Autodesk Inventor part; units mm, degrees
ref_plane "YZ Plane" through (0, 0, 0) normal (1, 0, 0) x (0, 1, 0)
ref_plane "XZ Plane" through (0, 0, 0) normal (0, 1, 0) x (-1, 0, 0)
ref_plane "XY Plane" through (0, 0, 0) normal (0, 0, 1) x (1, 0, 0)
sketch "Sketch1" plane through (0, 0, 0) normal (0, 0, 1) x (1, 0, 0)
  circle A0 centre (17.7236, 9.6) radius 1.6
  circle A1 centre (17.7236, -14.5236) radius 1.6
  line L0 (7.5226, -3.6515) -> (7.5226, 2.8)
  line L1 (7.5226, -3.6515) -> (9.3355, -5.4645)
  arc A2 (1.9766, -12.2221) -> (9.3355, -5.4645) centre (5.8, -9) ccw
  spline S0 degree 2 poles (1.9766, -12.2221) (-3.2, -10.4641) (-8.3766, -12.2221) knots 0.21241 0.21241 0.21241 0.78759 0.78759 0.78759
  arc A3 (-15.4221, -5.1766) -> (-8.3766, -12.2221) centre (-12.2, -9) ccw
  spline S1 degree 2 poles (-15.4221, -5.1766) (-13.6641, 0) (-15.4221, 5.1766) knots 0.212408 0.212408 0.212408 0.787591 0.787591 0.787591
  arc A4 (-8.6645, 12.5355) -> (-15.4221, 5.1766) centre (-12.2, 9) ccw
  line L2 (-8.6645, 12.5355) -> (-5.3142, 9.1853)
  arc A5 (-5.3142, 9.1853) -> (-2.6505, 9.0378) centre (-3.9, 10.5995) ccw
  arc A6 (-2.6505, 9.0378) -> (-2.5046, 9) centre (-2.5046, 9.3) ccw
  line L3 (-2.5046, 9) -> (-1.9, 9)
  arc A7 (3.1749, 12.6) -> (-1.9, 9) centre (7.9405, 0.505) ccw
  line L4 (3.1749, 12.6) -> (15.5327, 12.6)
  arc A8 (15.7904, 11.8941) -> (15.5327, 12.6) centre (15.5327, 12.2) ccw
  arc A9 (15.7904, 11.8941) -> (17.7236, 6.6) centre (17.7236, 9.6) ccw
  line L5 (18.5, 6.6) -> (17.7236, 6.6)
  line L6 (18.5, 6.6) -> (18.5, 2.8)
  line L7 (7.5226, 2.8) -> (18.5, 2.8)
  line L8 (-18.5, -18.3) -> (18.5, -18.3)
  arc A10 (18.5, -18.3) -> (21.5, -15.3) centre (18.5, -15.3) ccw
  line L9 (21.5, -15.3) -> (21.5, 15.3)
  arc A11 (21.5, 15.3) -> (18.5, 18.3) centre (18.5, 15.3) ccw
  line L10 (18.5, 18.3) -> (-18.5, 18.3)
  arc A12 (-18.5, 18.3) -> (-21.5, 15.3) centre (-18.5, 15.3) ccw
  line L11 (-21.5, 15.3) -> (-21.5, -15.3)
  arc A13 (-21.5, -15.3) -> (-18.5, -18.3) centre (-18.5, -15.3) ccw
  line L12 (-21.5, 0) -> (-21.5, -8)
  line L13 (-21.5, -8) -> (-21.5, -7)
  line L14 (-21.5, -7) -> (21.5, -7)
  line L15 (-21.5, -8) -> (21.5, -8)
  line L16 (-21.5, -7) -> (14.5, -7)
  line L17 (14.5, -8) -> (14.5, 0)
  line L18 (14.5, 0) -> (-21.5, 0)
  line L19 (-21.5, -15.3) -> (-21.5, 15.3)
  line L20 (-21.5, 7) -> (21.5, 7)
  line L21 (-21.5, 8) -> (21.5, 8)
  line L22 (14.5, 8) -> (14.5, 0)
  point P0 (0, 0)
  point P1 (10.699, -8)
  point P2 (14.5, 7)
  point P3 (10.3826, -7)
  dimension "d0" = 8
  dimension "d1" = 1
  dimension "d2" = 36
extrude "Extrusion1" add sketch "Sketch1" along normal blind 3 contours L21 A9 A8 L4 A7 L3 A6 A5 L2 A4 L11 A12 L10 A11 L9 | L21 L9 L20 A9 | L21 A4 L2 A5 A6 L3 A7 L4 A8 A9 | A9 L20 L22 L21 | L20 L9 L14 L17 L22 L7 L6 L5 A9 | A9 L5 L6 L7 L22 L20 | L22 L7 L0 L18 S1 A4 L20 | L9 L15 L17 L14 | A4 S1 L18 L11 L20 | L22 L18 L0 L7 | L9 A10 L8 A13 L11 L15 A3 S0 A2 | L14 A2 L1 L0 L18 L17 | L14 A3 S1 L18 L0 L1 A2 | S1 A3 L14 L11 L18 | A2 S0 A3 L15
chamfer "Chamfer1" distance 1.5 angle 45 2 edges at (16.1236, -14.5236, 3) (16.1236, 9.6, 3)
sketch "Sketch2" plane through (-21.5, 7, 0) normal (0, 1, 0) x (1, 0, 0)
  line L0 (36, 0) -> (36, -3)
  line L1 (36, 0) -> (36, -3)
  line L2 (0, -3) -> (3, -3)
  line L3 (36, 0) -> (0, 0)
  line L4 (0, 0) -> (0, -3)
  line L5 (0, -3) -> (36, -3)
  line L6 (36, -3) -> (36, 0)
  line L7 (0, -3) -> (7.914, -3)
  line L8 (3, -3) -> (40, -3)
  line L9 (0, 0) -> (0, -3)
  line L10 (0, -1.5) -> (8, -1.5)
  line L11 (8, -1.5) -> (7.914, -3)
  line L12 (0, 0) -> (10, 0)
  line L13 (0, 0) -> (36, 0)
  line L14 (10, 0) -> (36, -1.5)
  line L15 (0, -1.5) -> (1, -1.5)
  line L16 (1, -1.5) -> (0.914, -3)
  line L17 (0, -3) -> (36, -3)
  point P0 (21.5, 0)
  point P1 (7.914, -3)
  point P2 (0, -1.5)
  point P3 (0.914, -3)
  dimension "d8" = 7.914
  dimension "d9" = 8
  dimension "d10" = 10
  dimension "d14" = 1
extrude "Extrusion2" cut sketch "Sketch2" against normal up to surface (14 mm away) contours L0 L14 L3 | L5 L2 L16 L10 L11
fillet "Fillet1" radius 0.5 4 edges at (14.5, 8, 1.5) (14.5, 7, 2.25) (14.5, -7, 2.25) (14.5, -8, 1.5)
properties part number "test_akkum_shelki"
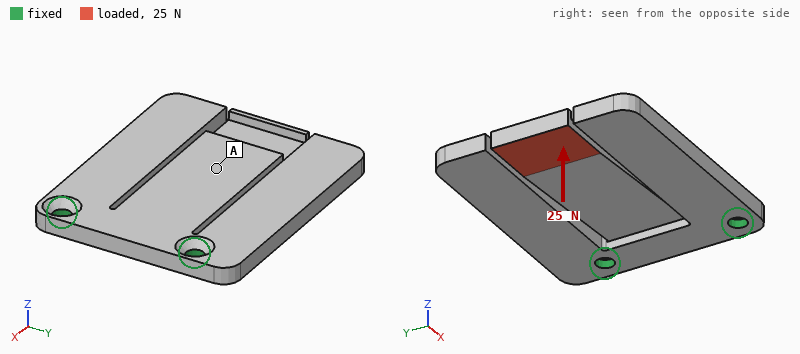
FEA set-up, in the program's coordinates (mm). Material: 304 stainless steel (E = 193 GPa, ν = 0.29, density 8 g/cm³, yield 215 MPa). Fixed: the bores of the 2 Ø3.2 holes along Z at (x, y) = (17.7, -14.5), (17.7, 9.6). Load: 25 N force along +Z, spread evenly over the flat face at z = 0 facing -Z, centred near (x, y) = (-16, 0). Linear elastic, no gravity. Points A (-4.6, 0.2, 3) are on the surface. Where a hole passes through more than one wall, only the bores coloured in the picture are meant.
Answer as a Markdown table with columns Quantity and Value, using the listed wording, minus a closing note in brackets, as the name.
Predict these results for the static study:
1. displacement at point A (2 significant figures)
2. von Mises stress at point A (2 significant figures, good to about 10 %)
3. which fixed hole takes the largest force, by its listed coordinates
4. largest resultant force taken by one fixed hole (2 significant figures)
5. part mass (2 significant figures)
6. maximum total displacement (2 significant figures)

| Quantity | Value |
|---|---|
| displacement at point A | 0.12 mm |
| von Mises stress at point A | 20 MPa |
| which fixed hole takes the largest force, by its listed coordinates | (17.7, 9.6) |
| largest resultant force taken by one fixed hole | 27 N |
| part mass | 32 g |
| maximum total displacement | 0.27 mm |
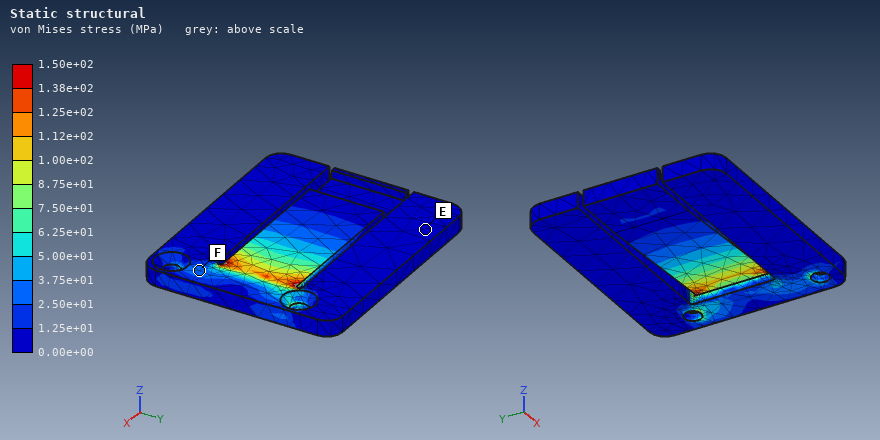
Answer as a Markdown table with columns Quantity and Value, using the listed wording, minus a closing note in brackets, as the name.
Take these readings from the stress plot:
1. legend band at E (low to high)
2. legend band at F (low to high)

| Quantity | Value |
|---|---|
| legend band at E | 0.00e+00 to 1.25e+01 MPa |
| legend band at F | 2.50e+01 to 3.75e+01 MPa |
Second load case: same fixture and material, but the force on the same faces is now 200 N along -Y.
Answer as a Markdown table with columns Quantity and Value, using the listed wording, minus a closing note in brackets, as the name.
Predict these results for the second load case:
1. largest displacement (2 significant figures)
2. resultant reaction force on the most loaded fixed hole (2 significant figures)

| Quantity | Value |
|---|---|
| largest displacement | 61 µm |
| resultant reaction force on the most loaded fixed hole | 360 N |
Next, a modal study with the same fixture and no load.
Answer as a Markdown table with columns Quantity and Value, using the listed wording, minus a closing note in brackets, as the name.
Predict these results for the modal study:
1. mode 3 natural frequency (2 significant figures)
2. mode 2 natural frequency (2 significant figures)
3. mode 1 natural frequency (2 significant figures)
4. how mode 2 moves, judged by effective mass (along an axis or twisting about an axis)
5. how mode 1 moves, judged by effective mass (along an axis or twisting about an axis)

| Quantity | Value |
|---|---|
| mode 3 natural frequency | 1500 Hz |
| mode 2 natural frequency | 1400 Hz |
| mode 1 natural frequency | 880 Hz |
| how mode 2 moves, judged by effective mass | along Z |
| how mode 1 moves, judged by effective mass | along Z |
